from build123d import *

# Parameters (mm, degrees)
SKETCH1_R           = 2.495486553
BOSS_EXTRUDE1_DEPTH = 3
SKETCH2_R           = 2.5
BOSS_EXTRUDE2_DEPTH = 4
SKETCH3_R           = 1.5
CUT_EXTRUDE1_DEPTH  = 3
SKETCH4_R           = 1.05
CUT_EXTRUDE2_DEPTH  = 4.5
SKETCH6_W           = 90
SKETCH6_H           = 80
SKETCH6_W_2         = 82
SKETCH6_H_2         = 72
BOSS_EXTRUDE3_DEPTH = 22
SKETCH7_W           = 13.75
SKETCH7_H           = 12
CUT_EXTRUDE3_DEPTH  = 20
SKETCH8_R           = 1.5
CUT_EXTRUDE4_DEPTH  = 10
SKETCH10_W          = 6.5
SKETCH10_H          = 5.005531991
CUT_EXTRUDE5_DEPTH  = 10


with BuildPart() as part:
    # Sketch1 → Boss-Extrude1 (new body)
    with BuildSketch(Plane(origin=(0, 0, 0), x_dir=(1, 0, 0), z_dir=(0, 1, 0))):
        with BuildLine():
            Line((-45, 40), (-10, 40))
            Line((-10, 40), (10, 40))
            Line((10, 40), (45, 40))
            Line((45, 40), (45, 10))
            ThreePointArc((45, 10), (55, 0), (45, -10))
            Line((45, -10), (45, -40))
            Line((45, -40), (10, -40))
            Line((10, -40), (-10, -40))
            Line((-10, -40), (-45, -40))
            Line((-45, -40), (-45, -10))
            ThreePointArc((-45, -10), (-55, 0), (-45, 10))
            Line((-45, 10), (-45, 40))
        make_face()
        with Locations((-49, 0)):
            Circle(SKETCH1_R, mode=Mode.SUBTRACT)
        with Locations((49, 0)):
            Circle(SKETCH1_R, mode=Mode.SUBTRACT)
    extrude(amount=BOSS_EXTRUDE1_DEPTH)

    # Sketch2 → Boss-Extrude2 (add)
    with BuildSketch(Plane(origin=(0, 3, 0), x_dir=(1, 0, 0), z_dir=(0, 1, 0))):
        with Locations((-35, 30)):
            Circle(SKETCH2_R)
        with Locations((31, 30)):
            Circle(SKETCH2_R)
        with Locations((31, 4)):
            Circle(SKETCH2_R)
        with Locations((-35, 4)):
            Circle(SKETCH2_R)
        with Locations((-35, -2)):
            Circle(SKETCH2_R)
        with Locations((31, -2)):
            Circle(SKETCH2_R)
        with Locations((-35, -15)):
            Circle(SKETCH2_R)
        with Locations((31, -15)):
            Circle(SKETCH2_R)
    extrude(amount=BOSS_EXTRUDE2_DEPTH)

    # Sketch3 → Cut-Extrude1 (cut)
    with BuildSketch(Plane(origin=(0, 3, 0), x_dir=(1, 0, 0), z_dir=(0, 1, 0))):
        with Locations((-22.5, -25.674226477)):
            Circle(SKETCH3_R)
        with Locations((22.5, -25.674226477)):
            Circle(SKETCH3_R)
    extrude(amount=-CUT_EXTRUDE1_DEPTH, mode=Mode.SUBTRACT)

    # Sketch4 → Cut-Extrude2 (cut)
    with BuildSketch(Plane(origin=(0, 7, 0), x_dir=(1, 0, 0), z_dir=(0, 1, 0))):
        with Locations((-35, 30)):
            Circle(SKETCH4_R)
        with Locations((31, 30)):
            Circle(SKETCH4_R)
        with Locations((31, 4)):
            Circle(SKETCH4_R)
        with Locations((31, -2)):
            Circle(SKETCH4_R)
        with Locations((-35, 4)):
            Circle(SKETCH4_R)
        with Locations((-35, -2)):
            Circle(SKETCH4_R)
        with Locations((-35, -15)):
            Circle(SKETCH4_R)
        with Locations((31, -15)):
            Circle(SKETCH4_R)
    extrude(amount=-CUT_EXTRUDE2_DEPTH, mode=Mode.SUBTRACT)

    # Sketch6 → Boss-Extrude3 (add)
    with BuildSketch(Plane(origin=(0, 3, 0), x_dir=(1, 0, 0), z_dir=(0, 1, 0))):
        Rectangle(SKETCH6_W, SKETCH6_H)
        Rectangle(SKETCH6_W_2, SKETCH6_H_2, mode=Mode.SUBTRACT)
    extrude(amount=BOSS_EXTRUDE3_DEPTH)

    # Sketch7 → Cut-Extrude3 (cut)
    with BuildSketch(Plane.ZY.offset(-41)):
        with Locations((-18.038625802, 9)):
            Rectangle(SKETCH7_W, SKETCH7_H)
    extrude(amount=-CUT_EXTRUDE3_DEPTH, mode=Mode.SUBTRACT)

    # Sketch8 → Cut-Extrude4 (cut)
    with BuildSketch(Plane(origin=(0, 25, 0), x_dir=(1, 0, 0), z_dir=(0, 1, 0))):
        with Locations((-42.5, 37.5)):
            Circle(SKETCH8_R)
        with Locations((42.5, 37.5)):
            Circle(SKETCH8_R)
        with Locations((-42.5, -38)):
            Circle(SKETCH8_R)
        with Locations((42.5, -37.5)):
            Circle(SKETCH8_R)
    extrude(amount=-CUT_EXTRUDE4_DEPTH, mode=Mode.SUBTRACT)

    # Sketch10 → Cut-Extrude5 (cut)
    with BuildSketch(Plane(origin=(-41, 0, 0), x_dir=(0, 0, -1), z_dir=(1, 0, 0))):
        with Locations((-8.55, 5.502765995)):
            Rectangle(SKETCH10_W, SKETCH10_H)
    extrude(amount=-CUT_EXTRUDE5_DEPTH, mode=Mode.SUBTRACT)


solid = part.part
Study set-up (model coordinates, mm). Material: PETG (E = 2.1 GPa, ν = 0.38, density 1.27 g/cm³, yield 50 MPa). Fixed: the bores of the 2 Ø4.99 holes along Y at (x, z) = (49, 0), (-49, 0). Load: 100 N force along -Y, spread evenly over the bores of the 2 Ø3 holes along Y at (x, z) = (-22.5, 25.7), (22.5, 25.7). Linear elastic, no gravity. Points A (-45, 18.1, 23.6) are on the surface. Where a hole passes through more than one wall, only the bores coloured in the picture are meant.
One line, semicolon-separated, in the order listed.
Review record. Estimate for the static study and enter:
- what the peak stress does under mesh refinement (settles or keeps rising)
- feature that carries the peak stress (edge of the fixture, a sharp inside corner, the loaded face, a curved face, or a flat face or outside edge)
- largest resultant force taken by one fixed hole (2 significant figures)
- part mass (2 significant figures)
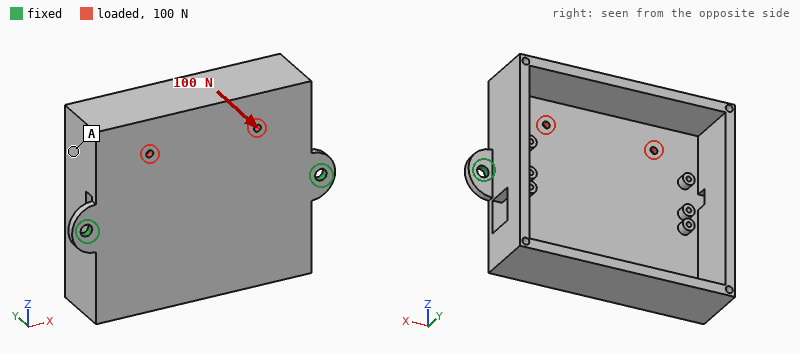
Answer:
keeps rising; edge of the fixture; 51 N; 64 g
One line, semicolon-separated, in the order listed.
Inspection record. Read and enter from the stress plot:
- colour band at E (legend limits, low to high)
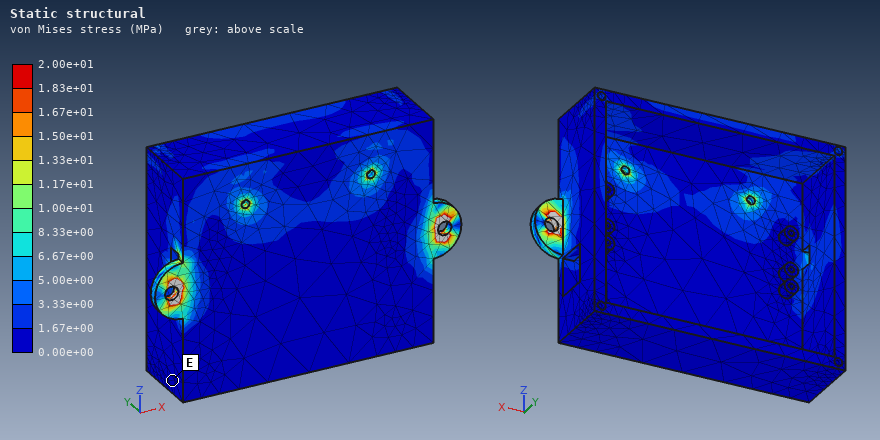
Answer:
0.00e+00 to 1.67e+00 MPa
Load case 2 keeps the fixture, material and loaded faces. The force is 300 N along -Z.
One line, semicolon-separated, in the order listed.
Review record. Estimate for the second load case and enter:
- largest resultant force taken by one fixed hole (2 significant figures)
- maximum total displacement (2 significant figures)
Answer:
150 N; 69 µm
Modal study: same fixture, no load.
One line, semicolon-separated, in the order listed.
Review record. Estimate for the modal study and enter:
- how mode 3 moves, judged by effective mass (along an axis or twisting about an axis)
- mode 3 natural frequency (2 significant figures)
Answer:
along Y; 660 Hz
